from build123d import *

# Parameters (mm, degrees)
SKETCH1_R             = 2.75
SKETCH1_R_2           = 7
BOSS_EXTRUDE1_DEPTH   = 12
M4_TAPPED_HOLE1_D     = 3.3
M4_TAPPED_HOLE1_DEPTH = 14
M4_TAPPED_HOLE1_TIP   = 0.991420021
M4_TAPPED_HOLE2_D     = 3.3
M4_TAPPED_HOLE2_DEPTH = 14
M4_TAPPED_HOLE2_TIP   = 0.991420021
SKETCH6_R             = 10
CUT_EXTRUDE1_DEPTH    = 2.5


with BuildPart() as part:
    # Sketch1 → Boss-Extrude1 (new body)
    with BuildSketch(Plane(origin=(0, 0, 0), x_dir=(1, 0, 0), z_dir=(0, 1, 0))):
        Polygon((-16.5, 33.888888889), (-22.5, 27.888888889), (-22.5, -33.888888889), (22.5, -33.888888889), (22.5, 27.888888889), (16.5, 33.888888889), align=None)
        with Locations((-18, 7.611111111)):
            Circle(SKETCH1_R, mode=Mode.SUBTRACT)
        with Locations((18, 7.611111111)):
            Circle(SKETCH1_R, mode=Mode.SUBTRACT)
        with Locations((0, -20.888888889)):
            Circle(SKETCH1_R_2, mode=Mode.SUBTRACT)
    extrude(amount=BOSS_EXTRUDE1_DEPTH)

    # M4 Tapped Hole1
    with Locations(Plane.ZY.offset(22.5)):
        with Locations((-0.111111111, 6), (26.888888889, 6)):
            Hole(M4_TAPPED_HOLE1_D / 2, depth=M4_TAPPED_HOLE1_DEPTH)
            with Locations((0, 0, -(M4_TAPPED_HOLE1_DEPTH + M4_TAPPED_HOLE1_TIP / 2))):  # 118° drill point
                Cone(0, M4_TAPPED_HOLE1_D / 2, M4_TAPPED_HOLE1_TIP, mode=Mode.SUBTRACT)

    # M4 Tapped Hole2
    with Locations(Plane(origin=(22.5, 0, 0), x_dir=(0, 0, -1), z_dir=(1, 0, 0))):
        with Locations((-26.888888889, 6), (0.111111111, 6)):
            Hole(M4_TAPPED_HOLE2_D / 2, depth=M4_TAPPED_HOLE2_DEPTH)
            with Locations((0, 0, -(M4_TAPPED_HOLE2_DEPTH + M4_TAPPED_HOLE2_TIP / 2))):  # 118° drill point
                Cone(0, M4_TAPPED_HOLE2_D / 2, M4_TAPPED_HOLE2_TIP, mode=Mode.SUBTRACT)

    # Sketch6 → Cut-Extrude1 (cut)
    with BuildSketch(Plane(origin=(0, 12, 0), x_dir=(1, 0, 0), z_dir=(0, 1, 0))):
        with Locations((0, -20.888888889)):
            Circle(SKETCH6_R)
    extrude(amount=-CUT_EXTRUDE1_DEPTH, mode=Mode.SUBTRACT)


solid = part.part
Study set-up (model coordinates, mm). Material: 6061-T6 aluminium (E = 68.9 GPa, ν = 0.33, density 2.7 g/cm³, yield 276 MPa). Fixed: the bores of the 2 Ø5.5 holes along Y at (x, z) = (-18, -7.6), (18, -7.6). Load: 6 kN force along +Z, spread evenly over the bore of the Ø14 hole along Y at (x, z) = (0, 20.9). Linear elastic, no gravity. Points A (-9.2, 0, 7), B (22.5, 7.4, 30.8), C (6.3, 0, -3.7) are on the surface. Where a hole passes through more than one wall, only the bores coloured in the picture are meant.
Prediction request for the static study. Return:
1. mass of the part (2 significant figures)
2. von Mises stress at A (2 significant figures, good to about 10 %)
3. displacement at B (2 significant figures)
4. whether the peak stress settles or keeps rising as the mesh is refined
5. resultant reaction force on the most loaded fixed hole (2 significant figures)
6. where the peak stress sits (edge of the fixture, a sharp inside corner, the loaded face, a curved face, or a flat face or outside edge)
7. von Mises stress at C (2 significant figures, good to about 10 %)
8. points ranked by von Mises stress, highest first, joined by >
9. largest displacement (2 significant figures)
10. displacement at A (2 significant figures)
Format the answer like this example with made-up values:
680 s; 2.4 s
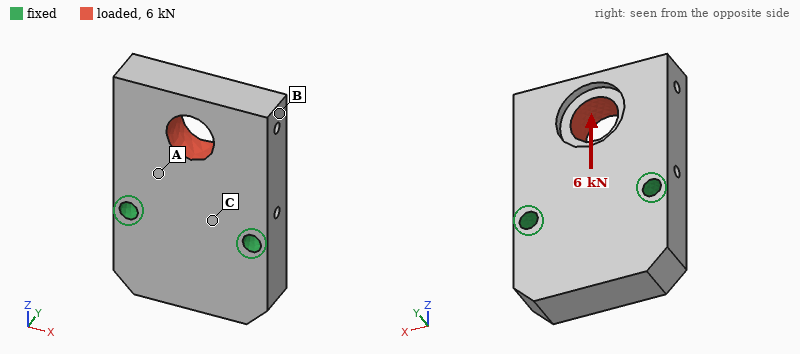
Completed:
89 g; 21 MPa; 12 µm; keeps rising; 3.0 kN; edge of the fixture; 11 MPa; A > C > B; 22 µm; 6.2 µm
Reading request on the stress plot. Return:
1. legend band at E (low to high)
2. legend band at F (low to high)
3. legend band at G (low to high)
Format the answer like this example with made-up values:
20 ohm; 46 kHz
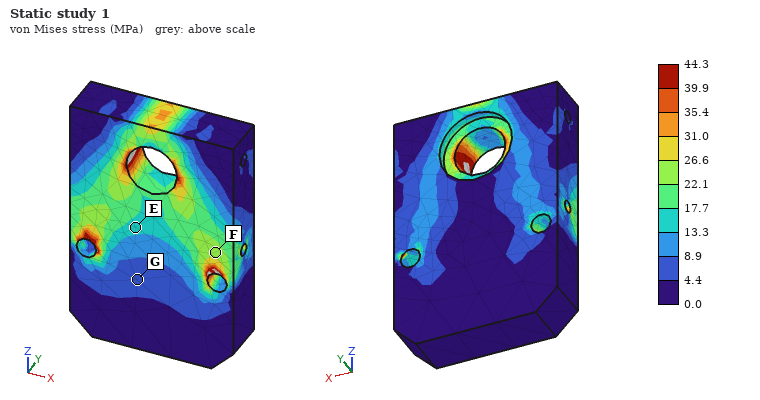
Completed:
13.3 to 17.7 MPa; 22.1 to 26.6 MPa; 4.4 to 8.9 MPa
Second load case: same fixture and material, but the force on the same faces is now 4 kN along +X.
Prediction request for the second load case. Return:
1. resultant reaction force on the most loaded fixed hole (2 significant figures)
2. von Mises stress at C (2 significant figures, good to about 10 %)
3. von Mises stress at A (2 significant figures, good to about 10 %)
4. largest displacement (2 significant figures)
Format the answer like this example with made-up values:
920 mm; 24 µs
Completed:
3.6 kN; 13 MPa; 18 MPa; 28 µm
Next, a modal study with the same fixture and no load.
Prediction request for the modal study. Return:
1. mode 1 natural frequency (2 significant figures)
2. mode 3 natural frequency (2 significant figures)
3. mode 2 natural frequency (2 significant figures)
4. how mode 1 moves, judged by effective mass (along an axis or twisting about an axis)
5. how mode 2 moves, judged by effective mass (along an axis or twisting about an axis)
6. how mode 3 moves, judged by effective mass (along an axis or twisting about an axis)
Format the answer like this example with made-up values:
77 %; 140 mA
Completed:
5200 Hz; 12 kHz; 9900 Hz; along Y; twisting about Z; along Y
